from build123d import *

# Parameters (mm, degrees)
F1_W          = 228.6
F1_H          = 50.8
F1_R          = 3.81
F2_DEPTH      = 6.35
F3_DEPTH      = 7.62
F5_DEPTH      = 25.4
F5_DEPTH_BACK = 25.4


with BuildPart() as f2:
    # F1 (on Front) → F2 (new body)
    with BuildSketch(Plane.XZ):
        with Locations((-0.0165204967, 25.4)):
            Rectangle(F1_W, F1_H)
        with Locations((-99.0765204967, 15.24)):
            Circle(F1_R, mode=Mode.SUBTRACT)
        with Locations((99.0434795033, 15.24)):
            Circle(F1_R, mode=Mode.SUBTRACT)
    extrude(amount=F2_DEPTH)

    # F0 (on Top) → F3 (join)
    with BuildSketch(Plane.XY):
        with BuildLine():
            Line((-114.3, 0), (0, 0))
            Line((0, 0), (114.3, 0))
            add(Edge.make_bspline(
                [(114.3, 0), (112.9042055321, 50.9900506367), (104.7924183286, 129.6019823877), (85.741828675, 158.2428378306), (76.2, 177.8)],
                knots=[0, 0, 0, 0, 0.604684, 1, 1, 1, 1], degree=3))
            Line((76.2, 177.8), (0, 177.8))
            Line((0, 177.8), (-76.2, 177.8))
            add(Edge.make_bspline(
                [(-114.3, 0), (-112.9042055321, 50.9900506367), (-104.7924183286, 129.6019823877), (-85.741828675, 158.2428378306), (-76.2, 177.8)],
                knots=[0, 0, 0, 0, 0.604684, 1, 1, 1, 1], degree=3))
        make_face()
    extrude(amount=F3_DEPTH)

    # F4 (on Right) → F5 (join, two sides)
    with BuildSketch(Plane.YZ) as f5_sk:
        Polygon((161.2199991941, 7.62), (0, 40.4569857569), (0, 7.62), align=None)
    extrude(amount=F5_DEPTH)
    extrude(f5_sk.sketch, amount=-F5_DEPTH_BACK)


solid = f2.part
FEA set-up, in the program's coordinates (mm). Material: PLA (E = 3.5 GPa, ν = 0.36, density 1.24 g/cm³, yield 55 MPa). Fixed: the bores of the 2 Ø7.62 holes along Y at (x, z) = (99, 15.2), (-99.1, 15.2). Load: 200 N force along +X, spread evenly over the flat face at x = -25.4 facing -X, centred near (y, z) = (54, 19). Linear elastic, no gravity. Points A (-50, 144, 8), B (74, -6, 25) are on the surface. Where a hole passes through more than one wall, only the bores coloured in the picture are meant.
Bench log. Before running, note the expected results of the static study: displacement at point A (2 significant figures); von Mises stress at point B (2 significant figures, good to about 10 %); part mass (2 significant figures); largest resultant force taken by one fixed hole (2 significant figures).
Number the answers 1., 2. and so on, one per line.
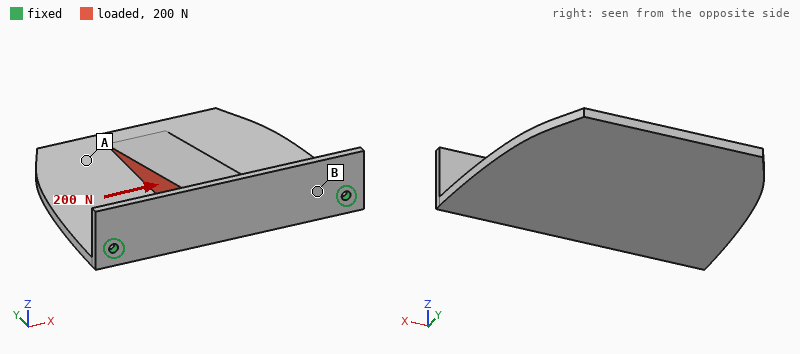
1. 29 µm
2. 0.28 MPa
3. 610 g
4. 120 N
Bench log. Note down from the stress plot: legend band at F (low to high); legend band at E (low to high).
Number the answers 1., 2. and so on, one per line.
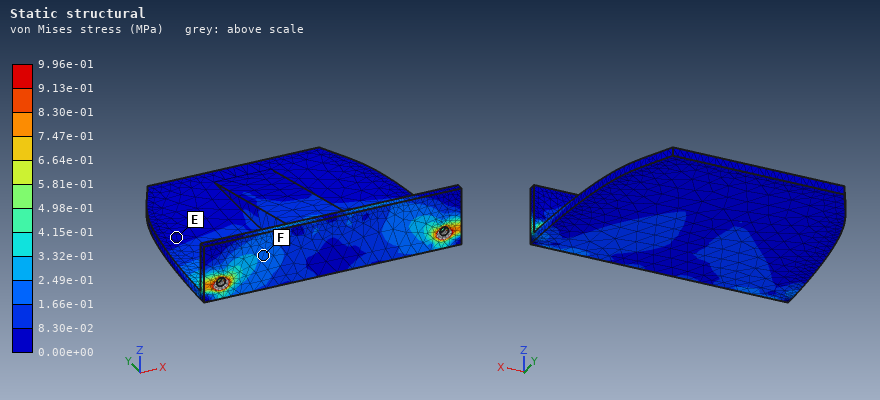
1. 1.66e-01 to 2.49e-01 MPa
2. 0.00e+00 to 8.30e-02 MPa
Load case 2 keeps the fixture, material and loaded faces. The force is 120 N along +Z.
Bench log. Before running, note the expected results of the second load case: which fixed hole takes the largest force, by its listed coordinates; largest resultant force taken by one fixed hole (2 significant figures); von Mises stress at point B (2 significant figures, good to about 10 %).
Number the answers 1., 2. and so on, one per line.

1. (-99.1, 15.2)
2. 76 N
3. 2.9 MPa
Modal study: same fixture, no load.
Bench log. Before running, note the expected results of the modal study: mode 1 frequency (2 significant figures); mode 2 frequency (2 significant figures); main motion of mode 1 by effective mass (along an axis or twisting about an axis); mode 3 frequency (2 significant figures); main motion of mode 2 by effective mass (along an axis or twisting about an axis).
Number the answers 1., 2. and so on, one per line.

1. 49 Hz
2. 280 Hz
3. along Z
4. 460 Hz
5. twisting about Y
